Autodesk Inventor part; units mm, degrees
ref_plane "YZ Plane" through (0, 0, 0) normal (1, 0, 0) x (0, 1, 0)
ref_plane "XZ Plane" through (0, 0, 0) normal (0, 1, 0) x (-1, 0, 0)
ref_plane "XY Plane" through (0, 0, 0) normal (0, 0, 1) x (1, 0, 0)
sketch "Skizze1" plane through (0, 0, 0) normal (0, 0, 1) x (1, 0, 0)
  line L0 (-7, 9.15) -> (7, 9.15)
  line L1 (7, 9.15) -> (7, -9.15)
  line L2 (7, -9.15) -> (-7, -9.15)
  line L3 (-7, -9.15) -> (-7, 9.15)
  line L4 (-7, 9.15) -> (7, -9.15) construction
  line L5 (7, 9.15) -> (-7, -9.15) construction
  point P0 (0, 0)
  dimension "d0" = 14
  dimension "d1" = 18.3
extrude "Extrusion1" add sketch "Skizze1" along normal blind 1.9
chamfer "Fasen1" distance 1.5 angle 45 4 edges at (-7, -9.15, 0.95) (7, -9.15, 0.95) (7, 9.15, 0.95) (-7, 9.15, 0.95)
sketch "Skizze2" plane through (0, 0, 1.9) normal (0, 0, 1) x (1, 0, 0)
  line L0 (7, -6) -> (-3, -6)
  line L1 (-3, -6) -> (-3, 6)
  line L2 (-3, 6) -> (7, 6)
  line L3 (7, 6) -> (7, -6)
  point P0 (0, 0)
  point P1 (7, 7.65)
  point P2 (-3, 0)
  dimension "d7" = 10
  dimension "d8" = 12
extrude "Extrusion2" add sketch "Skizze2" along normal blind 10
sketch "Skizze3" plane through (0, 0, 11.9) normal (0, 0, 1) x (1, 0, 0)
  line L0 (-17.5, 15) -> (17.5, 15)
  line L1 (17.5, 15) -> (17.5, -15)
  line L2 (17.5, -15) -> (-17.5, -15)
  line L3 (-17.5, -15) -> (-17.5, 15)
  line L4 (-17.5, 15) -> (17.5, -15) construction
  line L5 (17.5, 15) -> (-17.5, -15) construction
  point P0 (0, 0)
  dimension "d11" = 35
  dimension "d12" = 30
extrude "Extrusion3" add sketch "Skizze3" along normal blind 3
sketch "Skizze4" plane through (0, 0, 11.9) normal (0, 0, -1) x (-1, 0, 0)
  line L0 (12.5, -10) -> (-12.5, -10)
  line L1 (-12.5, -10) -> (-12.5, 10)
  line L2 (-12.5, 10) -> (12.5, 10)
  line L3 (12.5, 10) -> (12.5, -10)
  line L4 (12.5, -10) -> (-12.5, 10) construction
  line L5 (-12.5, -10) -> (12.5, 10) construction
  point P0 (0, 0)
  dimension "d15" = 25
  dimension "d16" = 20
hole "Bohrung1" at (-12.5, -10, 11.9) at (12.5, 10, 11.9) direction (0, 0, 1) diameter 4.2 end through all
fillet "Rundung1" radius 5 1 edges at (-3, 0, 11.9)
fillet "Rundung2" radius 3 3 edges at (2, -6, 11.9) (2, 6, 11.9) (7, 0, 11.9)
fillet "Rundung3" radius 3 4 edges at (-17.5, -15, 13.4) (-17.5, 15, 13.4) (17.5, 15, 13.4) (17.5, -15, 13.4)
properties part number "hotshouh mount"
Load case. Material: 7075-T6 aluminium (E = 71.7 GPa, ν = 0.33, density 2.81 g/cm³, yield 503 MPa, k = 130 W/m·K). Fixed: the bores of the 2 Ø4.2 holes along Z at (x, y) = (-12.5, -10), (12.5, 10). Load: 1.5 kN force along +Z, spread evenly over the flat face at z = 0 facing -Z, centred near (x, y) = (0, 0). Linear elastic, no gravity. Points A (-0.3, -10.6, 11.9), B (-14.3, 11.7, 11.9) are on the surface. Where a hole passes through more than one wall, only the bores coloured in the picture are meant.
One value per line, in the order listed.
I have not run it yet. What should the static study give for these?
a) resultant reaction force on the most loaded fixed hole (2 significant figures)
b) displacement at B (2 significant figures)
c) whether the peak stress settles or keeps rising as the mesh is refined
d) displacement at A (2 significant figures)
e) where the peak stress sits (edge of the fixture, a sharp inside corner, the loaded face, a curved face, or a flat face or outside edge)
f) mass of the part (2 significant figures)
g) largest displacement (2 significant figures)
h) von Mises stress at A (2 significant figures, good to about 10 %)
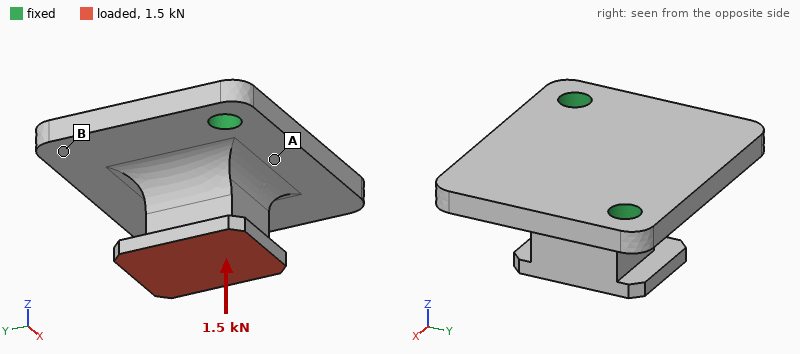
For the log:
860 N
36 µm
keeps rising
26 µm
edge of the fixture
14 g
59 µm
37 MPa
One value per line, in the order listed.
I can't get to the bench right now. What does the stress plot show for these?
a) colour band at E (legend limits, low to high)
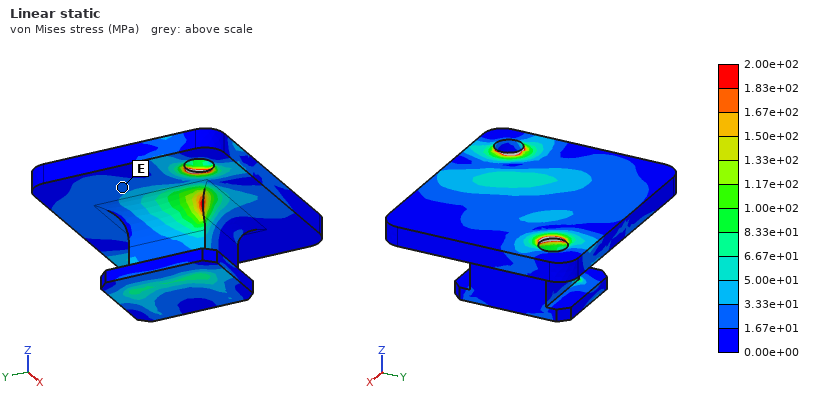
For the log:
1.67e+01 to 3.33e+01 MPa
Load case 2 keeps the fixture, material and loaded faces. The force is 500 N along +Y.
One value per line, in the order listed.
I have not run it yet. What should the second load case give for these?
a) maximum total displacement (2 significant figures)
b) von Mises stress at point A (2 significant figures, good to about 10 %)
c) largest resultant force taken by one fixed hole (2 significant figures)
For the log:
92 µm
31 MPa
300 N
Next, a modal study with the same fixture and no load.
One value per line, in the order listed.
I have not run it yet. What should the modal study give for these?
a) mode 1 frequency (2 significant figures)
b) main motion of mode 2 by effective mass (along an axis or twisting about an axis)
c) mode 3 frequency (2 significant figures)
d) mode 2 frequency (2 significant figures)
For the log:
5200 Hz
along Z
17 kHz
10000 Hz
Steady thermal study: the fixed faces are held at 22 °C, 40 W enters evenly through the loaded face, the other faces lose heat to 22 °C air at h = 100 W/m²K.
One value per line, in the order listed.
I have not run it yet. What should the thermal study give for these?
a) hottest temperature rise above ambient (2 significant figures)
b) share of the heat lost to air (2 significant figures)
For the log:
65 K
17 %
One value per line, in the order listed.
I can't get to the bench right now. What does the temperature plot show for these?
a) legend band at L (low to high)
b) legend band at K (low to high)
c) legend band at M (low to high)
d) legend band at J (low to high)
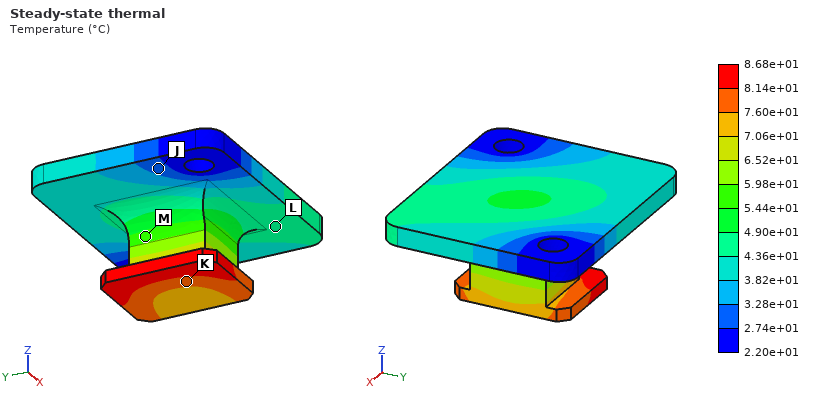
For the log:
4.36e+01 to 4.90e+01 °C
7.60e+01 to 8.14e+01 °C
5.44e+01 to 5.98e+01 °C
2.74e+01 to 3.28e+01 °C
